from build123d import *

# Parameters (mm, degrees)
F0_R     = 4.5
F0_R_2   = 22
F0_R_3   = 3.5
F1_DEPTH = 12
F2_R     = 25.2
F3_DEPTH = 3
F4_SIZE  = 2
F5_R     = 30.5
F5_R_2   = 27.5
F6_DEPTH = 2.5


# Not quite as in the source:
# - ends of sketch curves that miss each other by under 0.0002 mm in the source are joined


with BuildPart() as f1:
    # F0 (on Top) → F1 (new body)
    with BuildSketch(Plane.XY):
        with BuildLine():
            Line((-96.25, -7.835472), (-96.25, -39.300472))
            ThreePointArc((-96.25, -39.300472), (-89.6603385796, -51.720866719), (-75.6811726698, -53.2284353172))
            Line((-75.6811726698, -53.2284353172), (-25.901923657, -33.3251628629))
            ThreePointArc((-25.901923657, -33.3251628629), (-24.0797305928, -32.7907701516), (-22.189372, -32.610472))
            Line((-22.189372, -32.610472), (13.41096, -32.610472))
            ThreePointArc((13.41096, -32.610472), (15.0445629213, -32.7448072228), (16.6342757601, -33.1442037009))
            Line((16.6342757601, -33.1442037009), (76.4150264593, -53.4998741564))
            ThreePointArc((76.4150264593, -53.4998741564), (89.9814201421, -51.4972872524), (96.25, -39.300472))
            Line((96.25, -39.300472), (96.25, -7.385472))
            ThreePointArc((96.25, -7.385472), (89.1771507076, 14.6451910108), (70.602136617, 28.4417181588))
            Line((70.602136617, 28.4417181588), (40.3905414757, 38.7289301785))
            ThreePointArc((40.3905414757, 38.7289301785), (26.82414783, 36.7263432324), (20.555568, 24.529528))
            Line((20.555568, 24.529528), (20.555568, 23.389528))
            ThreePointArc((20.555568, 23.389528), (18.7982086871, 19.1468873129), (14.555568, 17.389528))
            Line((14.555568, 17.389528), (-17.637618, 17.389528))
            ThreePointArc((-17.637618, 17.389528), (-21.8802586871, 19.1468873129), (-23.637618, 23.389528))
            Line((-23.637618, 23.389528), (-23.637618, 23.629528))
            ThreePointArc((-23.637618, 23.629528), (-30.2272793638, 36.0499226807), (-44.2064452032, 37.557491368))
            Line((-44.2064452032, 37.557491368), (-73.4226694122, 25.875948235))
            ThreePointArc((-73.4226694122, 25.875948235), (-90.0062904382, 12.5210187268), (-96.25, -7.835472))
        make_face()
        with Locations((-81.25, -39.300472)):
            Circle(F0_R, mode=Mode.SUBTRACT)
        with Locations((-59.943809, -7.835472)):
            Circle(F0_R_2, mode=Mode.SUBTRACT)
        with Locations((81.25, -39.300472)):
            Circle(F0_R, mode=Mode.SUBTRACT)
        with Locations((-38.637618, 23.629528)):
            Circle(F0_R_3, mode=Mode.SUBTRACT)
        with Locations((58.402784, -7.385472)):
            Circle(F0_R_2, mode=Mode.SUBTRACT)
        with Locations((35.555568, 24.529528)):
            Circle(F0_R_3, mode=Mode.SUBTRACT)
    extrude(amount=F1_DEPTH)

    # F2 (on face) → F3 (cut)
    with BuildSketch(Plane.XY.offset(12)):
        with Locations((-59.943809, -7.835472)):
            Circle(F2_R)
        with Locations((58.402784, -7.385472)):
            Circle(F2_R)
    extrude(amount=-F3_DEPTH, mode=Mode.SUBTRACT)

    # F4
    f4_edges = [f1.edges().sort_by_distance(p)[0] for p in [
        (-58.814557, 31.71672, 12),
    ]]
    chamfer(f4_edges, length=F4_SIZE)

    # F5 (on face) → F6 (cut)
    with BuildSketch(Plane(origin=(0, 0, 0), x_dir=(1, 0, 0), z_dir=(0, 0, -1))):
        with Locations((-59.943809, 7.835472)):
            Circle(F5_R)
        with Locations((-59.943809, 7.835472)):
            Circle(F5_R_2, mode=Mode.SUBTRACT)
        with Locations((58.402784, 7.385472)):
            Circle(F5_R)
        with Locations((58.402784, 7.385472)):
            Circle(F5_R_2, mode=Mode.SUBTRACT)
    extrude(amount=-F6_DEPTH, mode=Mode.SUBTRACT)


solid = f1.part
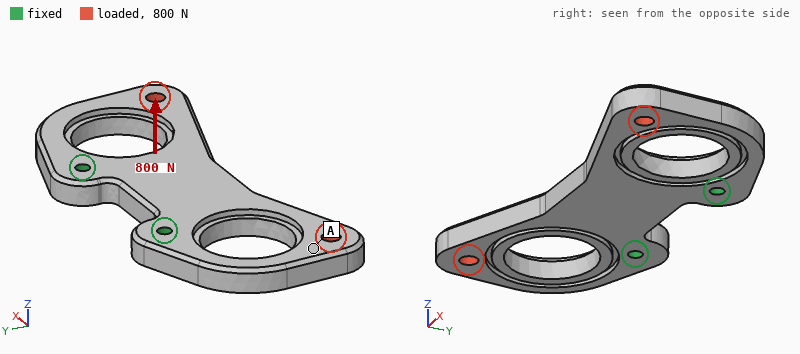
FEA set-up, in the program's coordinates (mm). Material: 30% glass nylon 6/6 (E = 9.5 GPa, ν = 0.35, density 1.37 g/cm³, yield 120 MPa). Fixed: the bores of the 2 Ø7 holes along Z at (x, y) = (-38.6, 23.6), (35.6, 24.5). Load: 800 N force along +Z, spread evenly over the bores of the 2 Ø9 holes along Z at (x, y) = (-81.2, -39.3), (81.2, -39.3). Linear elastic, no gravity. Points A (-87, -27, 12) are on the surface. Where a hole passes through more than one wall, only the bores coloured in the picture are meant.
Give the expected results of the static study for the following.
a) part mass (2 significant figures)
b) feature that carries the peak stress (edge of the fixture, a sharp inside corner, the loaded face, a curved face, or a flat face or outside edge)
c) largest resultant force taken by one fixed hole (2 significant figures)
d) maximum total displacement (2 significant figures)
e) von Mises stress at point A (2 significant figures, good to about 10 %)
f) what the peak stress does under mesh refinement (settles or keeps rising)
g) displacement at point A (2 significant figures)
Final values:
160 g
edge of the fixture
410 N
2.1 mm
5.9 MPa
keeps rising
1.4 mm
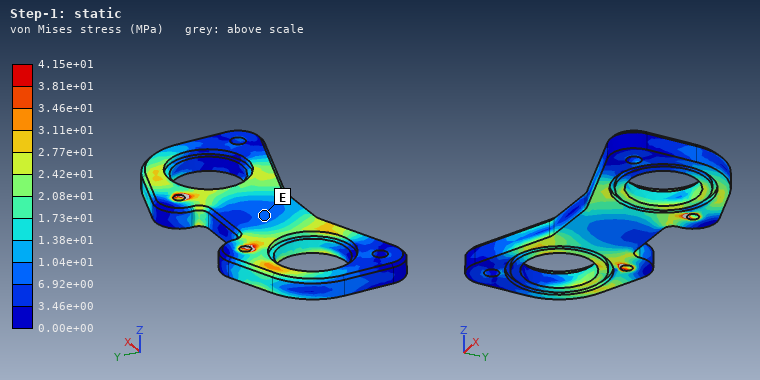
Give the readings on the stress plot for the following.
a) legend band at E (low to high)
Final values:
6.92e+00 to 1.04e+01 MPa
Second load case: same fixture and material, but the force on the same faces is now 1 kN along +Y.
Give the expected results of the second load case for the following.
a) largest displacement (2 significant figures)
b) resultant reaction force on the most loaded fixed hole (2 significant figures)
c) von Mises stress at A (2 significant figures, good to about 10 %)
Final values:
0.11 mm
640 N
1.8 MPa
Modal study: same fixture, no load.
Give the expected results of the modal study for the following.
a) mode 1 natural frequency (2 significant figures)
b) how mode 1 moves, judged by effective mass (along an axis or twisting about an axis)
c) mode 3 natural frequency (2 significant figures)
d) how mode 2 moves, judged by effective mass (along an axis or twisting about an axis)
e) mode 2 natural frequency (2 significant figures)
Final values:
550 Hz
along Z
1200 Hz
twisting about Y
610 Hz
